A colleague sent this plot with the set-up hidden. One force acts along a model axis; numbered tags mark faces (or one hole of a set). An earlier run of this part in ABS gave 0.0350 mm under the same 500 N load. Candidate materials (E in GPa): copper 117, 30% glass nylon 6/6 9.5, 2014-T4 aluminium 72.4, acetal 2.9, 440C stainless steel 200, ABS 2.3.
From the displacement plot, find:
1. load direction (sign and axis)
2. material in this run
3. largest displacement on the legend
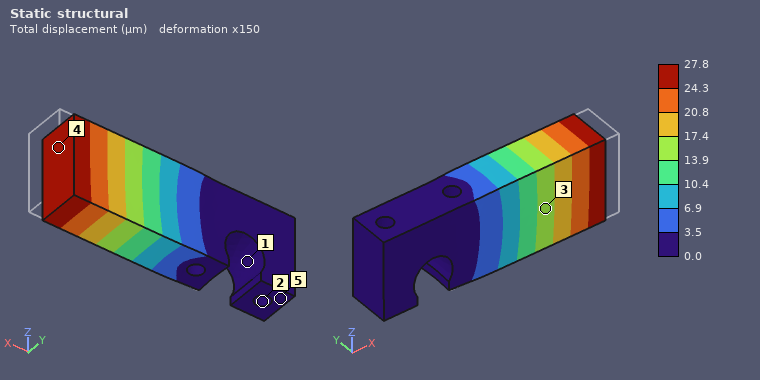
-X
acetal
27.8 µm
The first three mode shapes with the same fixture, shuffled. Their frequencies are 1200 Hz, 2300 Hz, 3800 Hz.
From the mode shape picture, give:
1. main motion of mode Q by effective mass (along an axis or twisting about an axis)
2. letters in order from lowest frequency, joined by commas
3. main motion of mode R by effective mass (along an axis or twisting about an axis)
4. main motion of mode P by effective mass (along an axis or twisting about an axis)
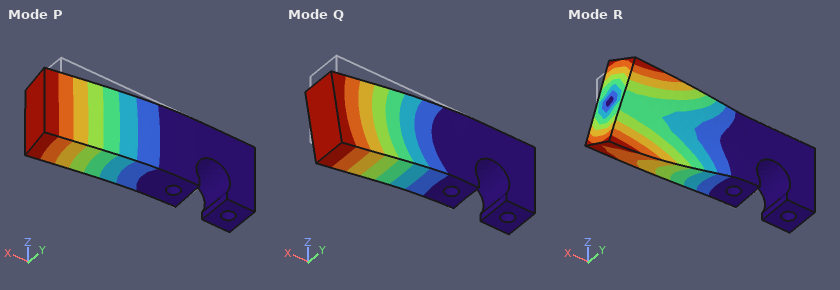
along Z
P, Q, R
twisting about X
along Y
